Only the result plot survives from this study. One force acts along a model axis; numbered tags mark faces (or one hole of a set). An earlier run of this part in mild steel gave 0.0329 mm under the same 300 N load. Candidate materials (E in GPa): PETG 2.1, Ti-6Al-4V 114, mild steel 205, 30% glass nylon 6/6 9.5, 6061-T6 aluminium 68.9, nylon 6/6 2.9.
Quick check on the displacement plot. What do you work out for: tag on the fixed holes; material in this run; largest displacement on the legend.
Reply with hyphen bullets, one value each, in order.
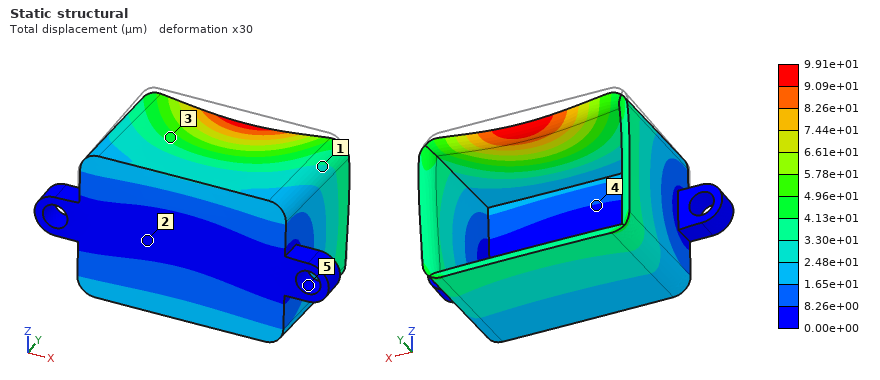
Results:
- 5
- 6061-T6 aluminium
- 9.91e+01 µm
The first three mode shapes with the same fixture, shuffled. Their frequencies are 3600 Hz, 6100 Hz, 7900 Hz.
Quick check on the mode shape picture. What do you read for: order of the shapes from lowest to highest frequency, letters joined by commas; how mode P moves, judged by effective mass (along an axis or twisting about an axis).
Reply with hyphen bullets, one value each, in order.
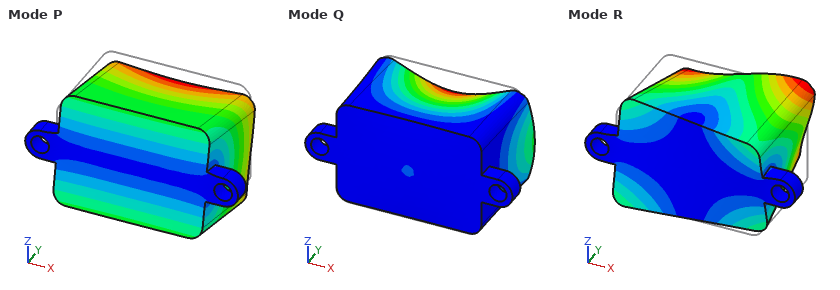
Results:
- P, R, Q
- along Z
